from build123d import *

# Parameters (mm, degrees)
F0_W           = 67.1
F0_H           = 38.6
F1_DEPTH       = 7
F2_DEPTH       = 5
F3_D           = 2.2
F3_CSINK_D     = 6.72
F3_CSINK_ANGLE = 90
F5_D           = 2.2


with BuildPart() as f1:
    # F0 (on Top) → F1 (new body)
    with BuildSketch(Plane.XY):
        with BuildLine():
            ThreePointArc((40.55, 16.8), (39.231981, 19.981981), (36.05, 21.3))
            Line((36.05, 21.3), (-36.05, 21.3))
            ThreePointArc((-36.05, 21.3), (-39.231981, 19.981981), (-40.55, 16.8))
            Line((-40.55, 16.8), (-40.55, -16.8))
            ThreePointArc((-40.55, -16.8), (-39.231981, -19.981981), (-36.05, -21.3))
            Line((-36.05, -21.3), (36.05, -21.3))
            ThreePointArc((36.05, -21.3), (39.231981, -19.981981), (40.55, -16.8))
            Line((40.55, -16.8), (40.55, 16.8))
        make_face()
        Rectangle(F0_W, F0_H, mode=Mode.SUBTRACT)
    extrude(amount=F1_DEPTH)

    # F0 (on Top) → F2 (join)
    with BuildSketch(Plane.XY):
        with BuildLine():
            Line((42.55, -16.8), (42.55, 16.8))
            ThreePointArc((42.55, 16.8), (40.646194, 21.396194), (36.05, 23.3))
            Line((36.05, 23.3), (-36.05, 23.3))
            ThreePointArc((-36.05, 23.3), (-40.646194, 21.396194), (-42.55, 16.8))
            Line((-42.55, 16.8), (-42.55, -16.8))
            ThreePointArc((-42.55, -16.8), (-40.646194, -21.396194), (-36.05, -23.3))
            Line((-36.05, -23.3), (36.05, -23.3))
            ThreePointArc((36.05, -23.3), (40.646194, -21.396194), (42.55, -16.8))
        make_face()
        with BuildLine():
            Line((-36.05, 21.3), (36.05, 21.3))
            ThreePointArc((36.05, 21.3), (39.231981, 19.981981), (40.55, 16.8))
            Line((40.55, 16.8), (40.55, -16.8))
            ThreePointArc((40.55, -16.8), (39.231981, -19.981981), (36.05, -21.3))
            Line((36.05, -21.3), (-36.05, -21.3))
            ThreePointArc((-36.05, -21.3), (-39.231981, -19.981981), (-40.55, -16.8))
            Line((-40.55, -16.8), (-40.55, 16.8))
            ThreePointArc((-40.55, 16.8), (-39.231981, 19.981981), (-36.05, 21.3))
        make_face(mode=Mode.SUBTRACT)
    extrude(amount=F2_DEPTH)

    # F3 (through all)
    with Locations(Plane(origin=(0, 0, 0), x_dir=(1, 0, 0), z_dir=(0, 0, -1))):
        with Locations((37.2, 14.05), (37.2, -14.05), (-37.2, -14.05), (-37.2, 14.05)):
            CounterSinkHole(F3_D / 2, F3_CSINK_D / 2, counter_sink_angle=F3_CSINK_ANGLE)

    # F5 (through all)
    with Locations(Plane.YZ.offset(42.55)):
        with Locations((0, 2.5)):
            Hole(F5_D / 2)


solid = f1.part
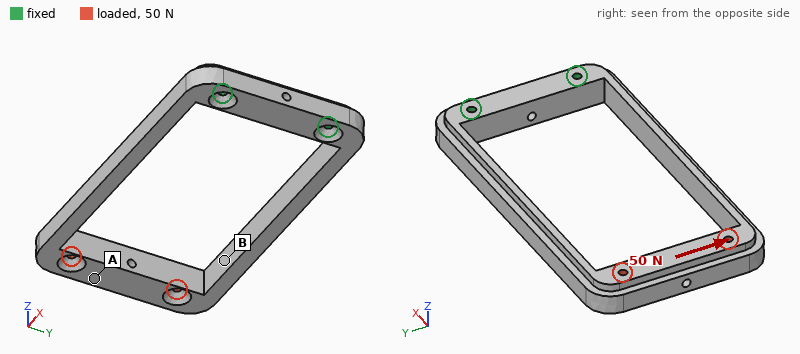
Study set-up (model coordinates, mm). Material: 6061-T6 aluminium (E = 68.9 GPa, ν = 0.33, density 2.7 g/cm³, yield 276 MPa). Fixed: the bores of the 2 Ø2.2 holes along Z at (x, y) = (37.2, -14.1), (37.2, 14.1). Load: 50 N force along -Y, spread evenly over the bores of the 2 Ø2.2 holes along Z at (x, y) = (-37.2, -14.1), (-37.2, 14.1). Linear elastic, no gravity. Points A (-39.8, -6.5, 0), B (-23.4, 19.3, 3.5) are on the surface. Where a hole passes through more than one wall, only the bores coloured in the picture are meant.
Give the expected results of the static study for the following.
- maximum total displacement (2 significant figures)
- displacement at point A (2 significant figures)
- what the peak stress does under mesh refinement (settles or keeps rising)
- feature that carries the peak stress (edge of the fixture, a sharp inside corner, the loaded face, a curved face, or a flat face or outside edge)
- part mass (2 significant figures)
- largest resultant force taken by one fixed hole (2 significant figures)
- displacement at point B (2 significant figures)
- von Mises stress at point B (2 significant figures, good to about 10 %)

0.41 mm
0.41 mm
keeps rising
edge of the fixture
22 g
100 N
0.37 mm
37 MPa
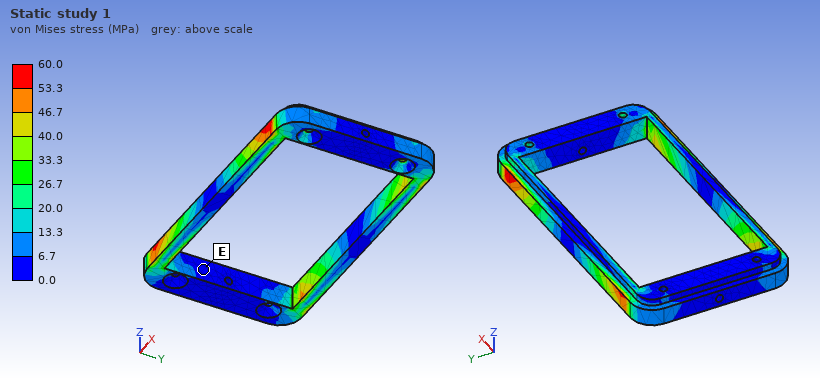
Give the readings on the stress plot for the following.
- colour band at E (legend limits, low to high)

0.0 to 6.7 MPa
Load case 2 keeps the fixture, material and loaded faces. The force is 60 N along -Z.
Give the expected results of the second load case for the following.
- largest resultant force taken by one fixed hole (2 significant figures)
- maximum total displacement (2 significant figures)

39 N
0.90 mm
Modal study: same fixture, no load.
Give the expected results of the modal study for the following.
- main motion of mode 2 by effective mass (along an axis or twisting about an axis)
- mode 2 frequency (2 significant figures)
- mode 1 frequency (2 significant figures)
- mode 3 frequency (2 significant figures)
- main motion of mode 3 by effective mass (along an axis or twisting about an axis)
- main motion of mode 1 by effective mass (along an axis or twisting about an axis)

along Y
560 Hz
460 Hz
1200 Hz
twisting about X
along Z
